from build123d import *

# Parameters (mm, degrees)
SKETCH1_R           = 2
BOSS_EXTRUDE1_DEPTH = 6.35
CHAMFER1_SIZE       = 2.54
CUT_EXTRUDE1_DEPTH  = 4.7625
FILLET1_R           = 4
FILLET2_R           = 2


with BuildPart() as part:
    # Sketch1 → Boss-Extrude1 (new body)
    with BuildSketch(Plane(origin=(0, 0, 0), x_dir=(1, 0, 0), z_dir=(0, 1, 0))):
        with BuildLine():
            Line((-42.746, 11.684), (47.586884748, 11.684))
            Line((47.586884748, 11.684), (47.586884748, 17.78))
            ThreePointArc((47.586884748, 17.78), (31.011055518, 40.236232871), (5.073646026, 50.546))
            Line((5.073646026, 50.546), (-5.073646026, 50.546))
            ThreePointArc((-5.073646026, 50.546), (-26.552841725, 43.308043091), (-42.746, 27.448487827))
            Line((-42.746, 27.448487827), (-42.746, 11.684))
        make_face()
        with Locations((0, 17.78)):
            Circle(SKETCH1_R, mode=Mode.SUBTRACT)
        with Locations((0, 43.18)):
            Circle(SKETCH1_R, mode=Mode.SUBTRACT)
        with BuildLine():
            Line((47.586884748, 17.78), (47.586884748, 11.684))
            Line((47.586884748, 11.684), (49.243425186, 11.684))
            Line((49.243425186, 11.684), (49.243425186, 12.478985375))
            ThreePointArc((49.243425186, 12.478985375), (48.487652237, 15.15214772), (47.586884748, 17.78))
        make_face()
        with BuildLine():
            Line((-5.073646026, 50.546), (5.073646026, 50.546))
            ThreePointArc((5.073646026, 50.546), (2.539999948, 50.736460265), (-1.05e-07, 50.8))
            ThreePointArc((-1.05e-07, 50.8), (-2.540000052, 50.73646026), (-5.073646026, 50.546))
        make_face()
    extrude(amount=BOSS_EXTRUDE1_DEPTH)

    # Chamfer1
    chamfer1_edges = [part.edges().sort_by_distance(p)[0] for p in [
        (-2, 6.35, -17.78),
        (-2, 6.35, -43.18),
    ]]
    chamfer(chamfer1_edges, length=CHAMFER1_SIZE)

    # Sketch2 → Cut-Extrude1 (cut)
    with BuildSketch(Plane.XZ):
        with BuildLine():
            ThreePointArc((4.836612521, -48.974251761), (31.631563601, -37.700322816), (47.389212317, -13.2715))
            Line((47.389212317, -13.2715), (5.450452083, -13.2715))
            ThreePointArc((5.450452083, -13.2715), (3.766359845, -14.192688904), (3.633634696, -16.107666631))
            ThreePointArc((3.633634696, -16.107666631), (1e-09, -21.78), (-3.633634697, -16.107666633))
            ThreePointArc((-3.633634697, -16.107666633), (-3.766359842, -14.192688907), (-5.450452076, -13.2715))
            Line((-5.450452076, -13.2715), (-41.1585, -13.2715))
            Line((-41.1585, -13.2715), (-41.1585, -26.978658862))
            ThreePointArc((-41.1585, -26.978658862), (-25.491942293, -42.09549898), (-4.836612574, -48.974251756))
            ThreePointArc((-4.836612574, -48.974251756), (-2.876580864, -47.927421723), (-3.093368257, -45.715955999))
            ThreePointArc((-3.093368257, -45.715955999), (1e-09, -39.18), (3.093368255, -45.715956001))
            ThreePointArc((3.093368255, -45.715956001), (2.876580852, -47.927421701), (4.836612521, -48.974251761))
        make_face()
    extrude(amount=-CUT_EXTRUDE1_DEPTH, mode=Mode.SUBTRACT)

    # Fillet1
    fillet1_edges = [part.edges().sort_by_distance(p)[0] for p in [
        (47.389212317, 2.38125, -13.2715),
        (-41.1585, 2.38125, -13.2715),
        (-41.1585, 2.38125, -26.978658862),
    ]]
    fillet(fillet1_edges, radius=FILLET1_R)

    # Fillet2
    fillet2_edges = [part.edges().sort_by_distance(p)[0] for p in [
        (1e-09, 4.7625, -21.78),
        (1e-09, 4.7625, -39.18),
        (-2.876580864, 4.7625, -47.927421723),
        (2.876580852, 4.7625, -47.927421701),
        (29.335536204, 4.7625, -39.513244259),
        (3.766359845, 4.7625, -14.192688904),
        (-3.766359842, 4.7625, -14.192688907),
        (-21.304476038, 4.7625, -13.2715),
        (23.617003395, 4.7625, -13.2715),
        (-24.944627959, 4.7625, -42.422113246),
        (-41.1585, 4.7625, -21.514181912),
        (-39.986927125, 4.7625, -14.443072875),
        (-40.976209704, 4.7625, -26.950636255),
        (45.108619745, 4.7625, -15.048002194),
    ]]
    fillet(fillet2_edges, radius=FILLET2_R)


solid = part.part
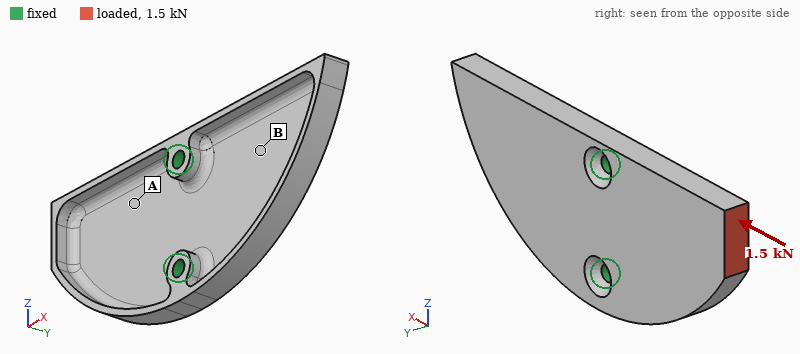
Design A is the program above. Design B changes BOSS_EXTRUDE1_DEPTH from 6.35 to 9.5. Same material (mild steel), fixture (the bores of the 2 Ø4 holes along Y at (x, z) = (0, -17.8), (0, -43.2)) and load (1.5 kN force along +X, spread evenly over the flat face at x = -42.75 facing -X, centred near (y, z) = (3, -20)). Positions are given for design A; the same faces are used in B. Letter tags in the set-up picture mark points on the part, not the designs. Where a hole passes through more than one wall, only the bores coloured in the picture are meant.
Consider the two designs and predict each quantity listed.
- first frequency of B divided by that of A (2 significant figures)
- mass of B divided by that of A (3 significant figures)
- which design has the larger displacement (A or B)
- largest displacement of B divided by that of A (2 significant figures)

1.5
2.31
A
0.27
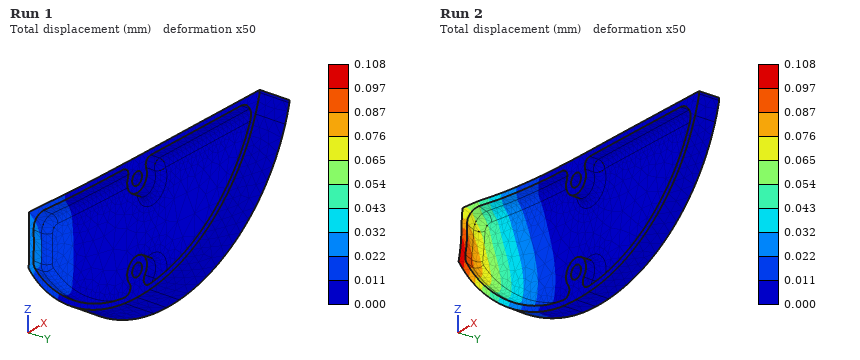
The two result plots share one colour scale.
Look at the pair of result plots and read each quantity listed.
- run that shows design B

Run 1
